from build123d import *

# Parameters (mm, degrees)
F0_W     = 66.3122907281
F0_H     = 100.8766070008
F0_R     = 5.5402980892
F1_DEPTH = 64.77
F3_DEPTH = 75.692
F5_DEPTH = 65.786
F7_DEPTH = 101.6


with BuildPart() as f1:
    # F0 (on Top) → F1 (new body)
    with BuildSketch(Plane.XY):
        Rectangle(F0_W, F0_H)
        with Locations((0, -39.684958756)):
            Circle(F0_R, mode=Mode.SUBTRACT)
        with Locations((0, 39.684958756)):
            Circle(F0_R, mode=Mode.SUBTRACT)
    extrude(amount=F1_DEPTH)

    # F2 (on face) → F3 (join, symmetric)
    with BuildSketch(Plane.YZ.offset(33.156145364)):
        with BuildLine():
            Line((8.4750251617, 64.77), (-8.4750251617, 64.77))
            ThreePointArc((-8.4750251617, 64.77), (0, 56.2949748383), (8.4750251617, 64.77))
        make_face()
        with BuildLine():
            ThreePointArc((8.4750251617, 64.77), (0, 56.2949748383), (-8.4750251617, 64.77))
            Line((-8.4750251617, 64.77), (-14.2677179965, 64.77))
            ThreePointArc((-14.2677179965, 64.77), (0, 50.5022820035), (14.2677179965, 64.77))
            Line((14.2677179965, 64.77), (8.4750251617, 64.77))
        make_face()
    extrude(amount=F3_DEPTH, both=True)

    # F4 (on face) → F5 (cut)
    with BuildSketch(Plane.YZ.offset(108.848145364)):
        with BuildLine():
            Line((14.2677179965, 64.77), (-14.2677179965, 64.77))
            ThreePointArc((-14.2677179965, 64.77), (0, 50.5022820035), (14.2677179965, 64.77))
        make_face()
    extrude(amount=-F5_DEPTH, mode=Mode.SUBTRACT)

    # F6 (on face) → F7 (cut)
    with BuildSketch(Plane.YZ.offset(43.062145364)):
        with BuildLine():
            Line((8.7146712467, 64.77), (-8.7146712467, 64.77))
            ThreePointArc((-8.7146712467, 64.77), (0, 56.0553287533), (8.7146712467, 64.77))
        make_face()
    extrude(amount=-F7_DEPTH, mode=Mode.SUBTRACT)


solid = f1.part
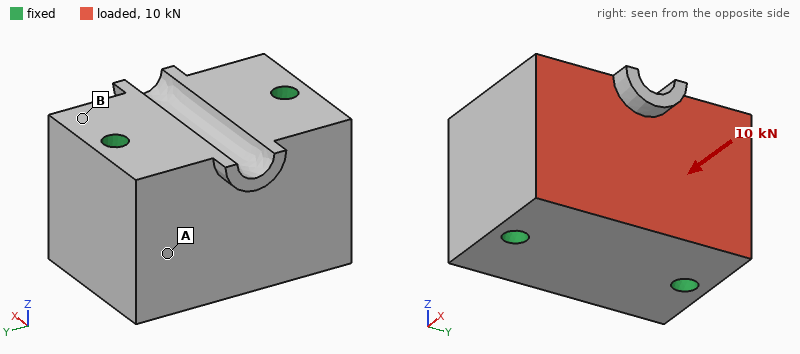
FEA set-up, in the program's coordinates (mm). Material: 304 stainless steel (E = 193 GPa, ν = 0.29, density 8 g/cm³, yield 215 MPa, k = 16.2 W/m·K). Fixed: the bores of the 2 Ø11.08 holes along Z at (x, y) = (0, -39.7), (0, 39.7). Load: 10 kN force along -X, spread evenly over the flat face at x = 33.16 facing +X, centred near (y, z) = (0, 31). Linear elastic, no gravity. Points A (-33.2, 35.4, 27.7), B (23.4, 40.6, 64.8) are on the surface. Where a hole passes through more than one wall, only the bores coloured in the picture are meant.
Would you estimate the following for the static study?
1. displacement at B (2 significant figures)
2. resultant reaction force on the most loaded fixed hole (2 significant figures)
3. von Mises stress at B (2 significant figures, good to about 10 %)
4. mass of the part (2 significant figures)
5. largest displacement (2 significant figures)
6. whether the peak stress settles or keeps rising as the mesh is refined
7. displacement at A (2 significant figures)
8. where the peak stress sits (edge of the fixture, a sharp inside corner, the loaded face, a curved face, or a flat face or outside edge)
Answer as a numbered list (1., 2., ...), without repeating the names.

1. 0.24 µm
2. 5.0 kN
3. 1.7 MPa
4. 3.3 kg
5. 0.65 µm
6. keeps rising
7. 0.18 µm
8. edge of the fixture
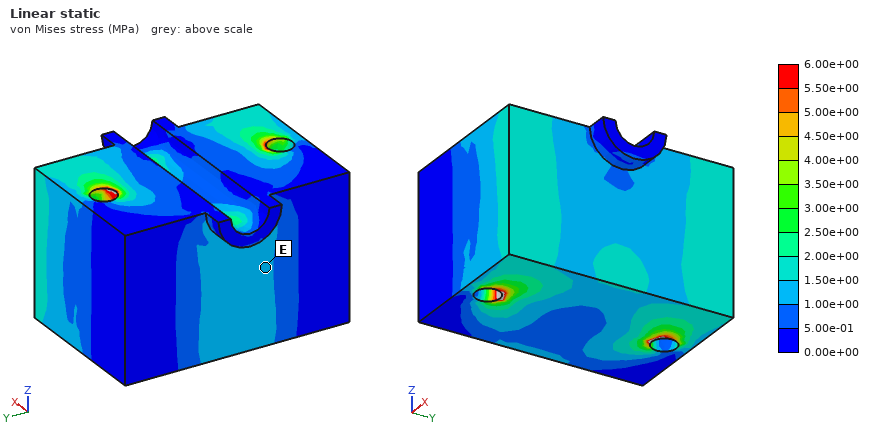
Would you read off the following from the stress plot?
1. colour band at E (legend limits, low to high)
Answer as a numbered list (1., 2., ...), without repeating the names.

1. 1.00e+00 to 1.50e+00 MPa
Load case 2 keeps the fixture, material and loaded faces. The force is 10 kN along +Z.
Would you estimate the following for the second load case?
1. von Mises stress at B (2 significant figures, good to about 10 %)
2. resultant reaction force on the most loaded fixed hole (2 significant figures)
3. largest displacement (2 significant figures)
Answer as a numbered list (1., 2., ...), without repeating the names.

1. 2.8 MPa
2. 5.0 kN
3. 2.2 µm
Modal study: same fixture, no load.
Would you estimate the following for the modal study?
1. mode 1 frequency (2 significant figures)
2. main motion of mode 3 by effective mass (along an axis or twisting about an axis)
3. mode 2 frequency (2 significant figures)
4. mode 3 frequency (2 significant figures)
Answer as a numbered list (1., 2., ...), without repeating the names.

1. 13 kHz
2. along X
3. 14 kHz
4. 14 kHz
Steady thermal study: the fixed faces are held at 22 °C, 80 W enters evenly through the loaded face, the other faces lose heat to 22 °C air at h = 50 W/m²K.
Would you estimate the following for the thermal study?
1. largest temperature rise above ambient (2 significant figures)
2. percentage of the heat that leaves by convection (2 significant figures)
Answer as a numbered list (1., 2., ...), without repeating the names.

1. 30 K
2. 15 %
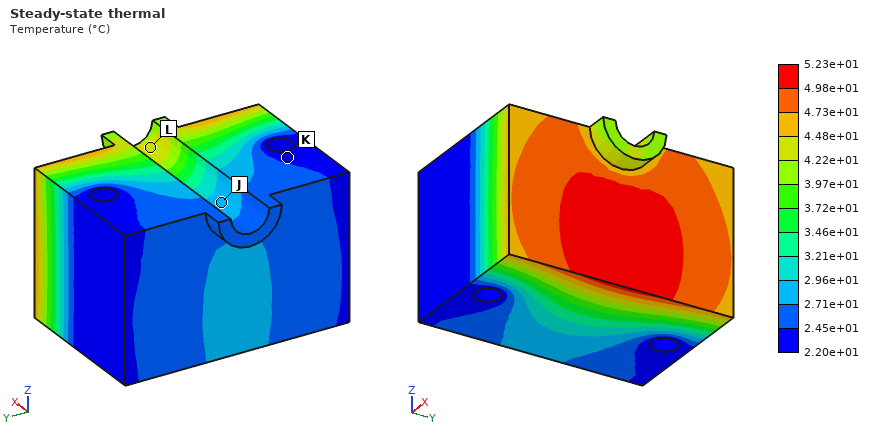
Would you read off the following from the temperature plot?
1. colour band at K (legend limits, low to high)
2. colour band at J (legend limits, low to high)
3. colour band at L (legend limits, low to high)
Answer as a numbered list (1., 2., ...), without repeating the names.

1. 2.20e+01 to 2.45e+01 °C
2. 2.71e+01 to 2.96e+01 °C
3. 4.22e+01 to 4.48e+01 °C
